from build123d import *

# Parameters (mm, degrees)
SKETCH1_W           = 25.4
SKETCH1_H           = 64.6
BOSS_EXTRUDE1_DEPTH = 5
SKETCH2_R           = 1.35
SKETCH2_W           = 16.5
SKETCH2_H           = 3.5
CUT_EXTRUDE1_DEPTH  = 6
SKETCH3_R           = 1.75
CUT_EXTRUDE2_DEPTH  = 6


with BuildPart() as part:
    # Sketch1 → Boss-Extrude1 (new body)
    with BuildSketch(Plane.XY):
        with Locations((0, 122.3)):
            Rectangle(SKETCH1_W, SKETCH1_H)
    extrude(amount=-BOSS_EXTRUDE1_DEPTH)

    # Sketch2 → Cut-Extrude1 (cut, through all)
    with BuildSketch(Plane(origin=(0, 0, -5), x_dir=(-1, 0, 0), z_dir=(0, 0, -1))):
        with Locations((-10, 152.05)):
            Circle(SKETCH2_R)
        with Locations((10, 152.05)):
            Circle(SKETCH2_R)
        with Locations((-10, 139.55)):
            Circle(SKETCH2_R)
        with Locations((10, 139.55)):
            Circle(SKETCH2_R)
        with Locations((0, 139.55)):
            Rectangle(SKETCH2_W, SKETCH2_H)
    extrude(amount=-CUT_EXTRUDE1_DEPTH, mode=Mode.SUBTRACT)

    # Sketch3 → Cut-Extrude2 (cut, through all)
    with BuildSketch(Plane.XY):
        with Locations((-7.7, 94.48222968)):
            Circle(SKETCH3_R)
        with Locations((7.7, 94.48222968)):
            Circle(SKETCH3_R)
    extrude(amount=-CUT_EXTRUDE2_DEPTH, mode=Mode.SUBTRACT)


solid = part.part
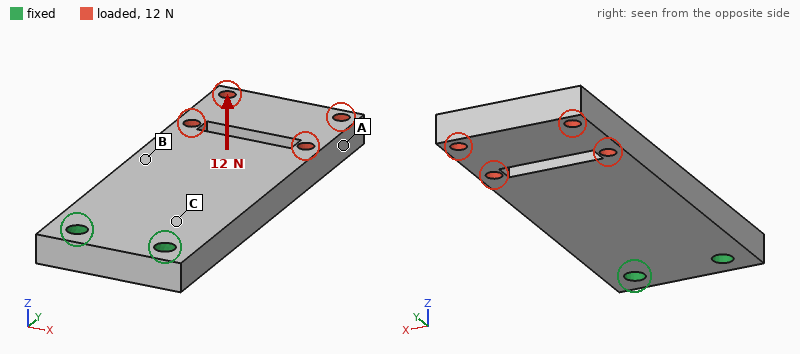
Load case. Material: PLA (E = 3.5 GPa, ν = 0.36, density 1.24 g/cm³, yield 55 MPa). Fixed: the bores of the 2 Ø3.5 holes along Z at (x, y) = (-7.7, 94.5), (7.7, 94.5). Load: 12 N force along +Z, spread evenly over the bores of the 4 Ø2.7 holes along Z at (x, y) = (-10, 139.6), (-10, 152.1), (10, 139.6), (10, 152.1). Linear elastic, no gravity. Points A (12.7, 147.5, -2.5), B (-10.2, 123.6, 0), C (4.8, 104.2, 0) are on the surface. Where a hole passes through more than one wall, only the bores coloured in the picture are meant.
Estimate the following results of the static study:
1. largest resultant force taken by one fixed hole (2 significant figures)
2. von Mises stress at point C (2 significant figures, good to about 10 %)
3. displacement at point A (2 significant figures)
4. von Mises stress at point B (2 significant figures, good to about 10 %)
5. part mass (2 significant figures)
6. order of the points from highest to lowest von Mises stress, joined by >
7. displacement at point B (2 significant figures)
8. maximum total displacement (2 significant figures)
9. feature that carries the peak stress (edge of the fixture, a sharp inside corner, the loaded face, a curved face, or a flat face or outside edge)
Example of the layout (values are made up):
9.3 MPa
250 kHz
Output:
6.0 N
4.4 MPa
0.63 mm
2.6 MPa
9.6 g
C > B > A
0.22 mm
0.77 mm
the loaded face
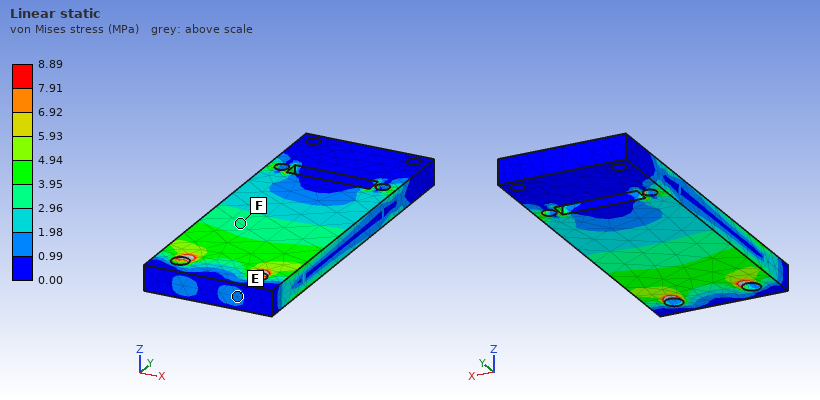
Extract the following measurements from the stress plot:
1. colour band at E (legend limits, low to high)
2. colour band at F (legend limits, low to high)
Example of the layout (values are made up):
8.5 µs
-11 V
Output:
0.99 to 1.98 MPa
2.96 to 3.95 MPa
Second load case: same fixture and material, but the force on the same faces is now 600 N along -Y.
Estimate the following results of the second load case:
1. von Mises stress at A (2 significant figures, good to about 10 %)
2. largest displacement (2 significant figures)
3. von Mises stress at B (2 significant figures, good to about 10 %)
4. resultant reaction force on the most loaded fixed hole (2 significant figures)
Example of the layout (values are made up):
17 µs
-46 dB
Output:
8.0 MPa
0.13 mm
6.0 MPa
300 N
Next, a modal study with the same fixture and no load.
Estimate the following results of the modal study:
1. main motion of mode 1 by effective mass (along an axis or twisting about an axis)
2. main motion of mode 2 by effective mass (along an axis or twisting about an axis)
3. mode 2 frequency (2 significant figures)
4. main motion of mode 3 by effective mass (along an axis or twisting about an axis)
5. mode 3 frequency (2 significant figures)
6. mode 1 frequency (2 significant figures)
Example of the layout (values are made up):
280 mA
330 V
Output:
along Z
along X
1600 Hz
twisting about Y
1700 Hz
390 Hz
